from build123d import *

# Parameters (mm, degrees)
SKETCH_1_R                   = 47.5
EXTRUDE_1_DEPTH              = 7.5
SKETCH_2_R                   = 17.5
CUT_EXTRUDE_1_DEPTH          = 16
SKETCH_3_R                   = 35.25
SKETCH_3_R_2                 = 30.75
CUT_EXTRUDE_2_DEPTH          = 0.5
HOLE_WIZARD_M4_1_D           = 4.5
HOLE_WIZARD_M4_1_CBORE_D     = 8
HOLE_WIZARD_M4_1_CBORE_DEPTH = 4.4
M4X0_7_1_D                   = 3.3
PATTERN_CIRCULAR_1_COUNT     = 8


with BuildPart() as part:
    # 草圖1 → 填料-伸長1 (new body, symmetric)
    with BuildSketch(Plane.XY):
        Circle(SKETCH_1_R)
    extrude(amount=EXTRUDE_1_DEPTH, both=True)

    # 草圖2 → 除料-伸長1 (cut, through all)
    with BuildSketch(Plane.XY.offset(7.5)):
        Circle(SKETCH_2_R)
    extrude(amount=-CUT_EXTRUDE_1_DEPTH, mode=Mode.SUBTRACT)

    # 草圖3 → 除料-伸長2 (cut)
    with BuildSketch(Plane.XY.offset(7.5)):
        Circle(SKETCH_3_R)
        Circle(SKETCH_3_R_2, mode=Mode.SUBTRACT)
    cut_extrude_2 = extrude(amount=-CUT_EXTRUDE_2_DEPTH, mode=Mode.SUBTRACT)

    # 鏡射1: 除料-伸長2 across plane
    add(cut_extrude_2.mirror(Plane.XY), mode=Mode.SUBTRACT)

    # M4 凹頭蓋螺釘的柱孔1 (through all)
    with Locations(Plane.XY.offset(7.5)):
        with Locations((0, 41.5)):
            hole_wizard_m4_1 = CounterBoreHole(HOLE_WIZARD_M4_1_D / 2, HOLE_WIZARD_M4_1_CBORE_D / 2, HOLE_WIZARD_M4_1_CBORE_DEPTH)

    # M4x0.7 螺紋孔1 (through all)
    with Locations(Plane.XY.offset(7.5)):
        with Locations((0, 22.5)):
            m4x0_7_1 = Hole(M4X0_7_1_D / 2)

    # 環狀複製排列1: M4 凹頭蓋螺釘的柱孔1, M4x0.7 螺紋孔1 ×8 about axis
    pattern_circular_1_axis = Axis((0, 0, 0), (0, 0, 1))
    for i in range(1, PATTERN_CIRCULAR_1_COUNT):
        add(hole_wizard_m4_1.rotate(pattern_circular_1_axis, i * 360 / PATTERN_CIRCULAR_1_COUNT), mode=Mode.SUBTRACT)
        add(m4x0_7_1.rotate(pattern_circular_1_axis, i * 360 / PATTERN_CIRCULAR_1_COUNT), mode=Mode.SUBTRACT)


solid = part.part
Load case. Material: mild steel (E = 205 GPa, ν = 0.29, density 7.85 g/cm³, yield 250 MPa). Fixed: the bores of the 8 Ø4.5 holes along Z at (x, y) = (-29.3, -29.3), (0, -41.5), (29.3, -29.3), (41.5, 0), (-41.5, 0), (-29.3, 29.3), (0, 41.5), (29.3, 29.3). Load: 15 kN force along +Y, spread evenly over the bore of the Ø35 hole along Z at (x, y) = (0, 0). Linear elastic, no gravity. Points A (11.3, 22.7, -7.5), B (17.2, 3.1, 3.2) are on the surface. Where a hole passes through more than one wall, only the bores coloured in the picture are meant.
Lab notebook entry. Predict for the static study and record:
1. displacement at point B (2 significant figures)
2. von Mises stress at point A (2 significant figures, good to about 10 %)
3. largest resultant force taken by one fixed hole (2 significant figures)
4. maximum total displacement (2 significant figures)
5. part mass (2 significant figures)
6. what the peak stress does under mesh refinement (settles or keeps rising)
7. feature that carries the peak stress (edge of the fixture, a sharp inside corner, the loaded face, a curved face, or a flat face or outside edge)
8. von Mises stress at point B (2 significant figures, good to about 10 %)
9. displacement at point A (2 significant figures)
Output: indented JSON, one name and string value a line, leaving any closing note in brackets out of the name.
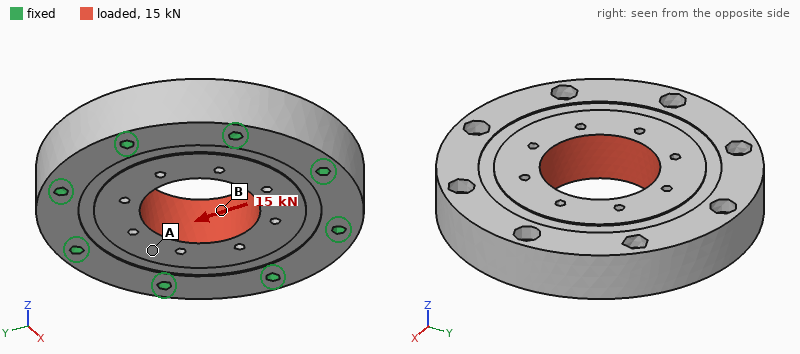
{
  "displacement at point B": "1.6 µm",
  "von Mises stress at point A": "7.8 MPa",
  "largest resultant force taken by one fixed hole": "2.8 kN",
  "maximum total displacement": "1.9 µm",
  "part mass": "680 g",
  "what the peak stress does under mesh refinement": "keeps rising",
  "feature that carries the peak stress": "edge of the fixture",
  "von Mises stress at point B": "15 MPa",
  "displacement at point A": "1.1 µm"
}
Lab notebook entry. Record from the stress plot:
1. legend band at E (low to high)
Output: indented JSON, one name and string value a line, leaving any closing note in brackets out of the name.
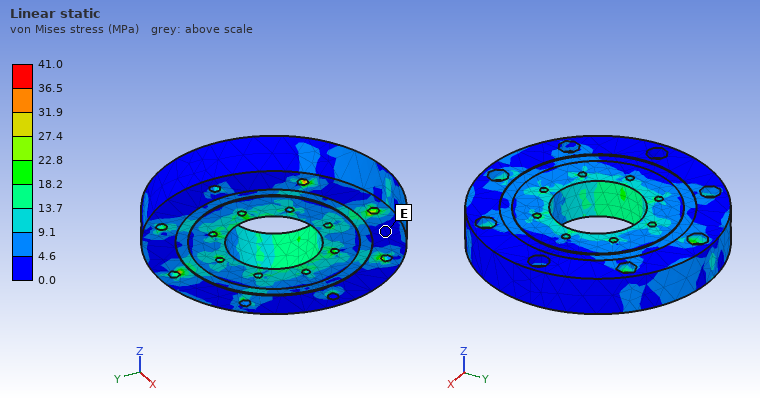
{
  "legend band at E": "0.0 to 4.6 MPa"
}
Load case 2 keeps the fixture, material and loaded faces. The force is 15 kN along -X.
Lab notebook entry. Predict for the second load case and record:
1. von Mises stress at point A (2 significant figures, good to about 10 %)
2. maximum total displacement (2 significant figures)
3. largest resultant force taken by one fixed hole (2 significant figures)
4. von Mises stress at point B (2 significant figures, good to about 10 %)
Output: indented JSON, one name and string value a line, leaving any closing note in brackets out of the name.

{
  "von Mises stress at point A": "9.1 MPa",
  "maximum total displacement": "1.9 µm",
  "largest resultant force taken by one fixed hole": "2.8 kN",
  "von Mises stress at point B": "9.2 MPa"
}
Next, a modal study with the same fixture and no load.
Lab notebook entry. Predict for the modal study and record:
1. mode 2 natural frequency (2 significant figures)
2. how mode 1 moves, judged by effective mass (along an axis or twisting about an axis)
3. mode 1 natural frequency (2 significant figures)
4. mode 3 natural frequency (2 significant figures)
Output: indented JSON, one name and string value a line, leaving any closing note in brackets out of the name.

{
  "mode 2 natural frequency": "21 kHz",
  "how mode 1 moves, judged by effective mass": "along Z",
  "mode 1 natural frequency": "15 kHz",
  "mode 3 natural frequency": "21 kHz"
}
